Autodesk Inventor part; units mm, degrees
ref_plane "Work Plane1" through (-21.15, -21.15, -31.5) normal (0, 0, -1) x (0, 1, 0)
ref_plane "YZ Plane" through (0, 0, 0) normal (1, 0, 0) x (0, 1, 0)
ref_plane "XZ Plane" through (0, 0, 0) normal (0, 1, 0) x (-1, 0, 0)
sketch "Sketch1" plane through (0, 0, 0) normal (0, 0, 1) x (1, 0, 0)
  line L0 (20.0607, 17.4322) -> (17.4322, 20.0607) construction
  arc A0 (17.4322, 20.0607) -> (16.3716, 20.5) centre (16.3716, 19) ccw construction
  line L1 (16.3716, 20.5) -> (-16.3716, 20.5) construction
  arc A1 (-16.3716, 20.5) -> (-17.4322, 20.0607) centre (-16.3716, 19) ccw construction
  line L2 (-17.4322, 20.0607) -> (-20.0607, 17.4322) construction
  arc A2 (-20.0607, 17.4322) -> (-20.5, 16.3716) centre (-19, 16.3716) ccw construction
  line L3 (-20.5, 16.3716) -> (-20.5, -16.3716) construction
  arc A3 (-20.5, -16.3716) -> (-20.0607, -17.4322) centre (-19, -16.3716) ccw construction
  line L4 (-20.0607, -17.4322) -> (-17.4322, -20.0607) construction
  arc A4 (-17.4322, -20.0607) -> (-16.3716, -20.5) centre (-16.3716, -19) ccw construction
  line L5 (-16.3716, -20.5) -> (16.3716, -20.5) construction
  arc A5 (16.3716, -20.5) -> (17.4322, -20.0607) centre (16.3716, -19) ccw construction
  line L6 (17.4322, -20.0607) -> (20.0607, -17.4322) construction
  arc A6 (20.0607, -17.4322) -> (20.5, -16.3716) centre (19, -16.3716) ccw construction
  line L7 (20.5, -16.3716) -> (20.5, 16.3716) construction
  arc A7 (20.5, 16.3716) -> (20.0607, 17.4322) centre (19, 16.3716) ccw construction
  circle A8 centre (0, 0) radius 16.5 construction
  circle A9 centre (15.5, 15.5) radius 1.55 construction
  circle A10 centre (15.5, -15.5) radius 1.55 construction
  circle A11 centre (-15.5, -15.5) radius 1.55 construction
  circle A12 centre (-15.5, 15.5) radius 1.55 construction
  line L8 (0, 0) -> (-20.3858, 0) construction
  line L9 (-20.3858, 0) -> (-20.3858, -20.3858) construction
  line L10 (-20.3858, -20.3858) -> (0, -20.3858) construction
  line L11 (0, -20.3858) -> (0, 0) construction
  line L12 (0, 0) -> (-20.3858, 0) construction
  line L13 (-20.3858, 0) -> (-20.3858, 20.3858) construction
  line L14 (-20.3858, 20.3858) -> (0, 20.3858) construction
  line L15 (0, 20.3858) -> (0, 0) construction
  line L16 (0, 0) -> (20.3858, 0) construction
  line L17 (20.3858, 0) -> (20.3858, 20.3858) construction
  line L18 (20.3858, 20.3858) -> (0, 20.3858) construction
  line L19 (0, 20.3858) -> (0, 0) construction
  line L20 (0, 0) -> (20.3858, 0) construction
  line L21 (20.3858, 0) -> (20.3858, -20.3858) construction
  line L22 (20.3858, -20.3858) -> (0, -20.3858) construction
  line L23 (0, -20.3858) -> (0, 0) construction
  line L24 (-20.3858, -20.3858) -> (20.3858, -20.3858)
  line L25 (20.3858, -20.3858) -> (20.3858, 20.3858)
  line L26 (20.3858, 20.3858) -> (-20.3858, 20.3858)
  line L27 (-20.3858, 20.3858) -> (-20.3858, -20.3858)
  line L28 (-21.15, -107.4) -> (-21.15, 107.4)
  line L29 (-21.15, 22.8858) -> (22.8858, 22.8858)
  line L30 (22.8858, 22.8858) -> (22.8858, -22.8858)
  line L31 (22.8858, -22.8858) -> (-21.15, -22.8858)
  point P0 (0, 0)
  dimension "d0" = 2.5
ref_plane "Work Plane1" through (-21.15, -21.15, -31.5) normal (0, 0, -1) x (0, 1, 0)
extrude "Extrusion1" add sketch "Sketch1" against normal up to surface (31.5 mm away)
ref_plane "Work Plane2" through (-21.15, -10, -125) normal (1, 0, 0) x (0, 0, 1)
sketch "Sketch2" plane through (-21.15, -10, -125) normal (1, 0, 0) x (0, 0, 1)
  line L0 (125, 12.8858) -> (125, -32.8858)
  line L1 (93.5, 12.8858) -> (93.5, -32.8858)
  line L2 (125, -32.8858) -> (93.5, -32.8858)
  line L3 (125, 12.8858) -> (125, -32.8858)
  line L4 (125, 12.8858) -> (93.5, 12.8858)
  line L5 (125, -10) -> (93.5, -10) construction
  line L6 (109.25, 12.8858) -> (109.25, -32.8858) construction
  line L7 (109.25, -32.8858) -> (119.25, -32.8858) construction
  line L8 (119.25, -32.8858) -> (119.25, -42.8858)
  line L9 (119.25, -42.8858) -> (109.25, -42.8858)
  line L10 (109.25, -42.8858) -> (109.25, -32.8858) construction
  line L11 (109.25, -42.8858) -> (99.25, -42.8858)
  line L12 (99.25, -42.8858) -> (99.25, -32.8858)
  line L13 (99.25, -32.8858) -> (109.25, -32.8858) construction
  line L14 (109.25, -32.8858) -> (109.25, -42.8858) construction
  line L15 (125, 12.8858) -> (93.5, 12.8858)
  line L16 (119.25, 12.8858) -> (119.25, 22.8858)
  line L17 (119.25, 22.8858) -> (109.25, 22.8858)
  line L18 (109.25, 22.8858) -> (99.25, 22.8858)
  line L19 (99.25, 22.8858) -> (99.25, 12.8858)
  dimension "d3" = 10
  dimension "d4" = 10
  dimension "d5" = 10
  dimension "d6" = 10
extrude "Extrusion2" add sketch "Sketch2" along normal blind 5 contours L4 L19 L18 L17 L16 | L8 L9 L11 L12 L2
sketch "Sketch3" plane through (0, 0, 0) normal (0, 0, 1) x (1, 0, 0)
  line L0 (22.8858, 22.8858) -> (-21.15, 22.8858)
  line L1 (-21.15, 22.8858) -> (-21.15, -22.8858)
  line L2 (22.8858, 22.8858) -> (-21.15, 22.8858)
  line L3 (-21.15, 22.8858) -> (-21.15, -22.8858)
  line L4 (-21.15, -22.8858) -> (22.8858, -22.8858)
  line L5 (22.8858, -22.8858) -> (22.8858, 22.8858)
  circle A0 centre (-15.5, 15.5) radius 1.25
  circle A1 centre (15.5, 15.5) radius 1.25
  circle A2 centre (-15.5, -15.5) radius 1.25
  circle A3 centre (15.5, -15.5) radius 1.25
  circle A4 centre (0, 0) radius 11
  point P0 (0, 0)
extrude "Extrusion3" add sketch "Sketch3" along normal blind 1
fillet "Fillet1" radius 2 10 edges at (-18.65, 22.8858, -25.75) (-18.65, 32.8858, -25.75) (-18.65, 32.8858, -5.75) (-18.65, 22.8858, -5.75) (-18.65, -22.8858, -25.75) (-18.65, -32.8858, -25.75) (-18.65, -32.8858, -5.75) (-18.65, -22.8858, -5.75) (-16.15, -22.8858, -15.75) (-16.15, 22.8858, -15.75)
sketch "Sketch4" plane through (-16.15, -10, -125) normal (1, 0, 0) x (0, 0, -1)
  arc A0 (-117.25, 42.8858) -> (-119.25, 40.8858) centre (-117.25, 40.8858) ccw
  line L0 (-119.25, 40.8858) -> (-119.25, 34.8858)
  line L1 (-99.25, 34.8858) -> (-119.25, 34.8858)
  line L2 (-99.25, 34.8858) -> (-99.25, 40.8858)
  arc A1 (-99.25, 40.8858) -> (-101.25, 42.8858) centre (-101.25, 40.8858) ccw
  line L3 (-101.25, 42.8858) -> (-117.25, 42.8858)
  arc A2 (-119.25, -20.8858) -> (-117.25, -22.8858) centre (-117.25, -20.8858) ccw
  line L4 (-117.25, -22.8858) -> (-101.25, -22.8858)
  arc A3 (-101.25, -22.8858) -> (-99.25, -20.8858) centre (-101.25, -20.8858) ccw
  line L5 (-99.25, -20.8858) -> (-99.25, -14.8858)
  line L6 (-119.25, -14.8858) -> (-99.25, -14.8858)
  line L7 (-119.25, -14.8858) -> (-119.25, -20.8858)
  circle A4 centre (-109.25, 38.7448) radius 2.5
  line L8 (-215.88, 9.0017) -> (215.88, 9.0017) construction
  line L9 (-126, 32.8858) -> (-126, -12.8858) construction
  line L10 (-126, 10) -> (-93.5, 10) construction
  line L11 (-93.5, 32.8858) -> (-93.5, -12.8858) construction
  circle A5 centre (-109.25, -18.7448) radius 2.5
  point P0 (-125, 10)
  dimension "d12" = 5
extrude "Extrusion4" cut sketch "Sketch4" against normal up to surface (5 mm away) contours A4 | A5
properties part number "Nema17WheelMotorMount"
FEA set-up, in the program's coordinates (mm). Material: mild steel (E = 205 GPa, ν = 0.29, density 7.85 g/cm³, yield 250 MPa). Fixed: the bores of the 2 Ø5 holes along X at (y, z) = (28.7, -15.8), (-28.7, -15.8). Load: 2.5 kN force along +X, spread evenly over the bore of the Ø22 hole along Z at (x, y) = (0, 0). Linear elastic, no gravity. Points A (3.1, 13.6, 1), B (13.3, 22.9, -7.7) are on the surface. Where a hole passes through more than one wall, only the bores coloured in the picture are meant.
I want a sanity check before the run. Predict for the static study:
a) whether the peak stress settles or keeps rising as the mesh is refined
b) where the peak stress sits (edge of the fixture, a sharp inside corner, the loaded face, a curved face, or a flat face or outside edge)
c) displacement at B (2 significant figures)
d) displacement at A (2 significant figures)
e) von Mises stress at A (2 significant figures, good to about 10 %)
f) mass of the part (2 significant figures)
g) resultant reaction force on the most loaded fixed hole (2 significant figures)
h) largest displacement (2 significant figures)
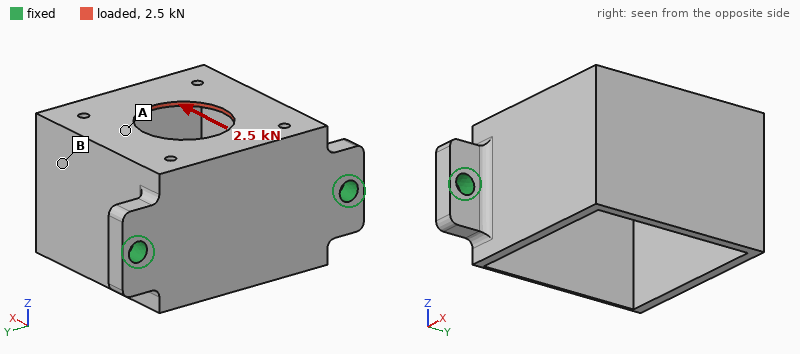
keeps rising
edge of the fixture
0.074 mm
0.067 mm
75 MPa
110 g
1.3 kN
0.10 mm
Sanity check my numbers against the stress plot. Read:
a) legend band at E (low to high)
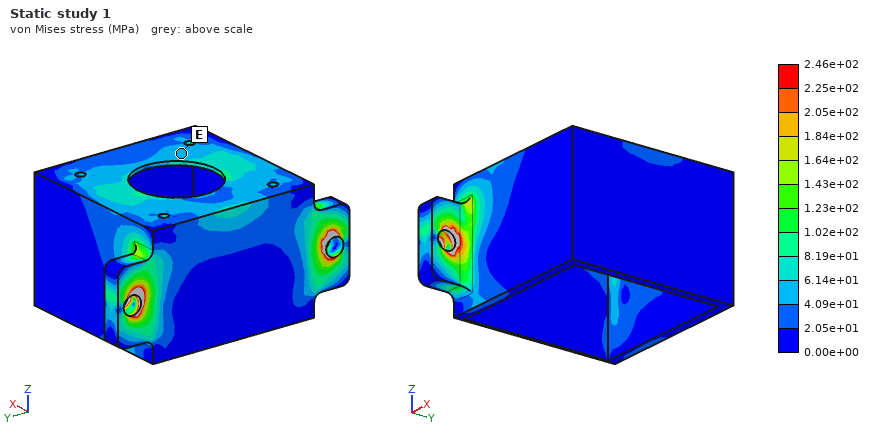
4.09e+01 to 6.14e+01 MPa
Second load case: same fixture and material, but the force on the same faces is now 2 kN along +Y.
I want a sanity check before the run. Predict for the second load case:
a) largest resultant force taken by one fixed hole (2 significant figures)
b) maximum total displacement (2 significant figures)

1.3 kN
96 µm
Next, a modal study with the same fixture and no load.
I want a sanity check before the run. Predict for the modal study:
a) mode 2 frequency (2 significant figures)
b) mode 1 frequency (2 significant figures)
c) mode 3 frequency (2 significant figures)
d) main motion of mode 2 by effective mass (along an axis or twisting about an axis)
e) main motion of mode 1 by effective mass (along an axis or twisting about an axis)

2300 Hz
1900 Hz
2700 Hz
along Z
along Y
